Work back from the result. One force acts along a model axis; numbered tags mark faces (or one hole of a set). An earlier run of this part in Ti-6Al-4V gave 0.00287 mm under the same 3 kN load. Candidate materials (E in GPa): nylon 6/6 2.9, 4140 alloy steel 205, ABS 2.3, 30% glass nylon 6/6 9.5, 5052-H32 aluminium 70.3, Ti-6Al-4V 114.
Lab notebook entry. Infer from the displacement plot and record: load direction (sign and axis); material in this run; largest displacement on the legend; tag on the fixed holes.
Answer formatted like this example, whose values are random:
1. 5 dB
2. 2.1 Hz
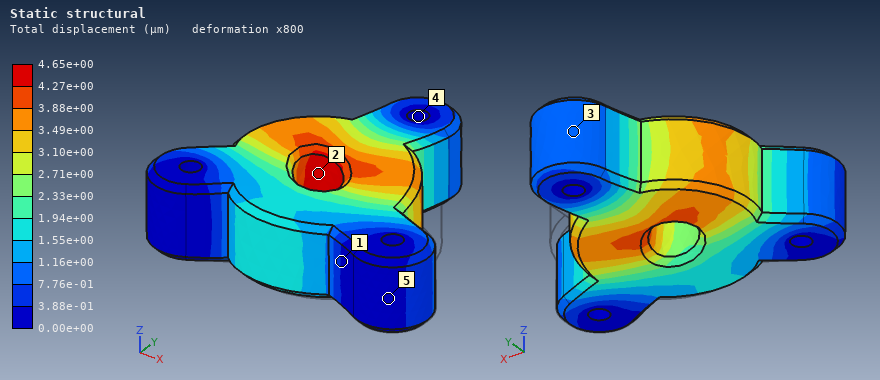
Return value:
1. -X
2. 5052-H32 aluminium
3. 4.65e+00 µm
4. 4
